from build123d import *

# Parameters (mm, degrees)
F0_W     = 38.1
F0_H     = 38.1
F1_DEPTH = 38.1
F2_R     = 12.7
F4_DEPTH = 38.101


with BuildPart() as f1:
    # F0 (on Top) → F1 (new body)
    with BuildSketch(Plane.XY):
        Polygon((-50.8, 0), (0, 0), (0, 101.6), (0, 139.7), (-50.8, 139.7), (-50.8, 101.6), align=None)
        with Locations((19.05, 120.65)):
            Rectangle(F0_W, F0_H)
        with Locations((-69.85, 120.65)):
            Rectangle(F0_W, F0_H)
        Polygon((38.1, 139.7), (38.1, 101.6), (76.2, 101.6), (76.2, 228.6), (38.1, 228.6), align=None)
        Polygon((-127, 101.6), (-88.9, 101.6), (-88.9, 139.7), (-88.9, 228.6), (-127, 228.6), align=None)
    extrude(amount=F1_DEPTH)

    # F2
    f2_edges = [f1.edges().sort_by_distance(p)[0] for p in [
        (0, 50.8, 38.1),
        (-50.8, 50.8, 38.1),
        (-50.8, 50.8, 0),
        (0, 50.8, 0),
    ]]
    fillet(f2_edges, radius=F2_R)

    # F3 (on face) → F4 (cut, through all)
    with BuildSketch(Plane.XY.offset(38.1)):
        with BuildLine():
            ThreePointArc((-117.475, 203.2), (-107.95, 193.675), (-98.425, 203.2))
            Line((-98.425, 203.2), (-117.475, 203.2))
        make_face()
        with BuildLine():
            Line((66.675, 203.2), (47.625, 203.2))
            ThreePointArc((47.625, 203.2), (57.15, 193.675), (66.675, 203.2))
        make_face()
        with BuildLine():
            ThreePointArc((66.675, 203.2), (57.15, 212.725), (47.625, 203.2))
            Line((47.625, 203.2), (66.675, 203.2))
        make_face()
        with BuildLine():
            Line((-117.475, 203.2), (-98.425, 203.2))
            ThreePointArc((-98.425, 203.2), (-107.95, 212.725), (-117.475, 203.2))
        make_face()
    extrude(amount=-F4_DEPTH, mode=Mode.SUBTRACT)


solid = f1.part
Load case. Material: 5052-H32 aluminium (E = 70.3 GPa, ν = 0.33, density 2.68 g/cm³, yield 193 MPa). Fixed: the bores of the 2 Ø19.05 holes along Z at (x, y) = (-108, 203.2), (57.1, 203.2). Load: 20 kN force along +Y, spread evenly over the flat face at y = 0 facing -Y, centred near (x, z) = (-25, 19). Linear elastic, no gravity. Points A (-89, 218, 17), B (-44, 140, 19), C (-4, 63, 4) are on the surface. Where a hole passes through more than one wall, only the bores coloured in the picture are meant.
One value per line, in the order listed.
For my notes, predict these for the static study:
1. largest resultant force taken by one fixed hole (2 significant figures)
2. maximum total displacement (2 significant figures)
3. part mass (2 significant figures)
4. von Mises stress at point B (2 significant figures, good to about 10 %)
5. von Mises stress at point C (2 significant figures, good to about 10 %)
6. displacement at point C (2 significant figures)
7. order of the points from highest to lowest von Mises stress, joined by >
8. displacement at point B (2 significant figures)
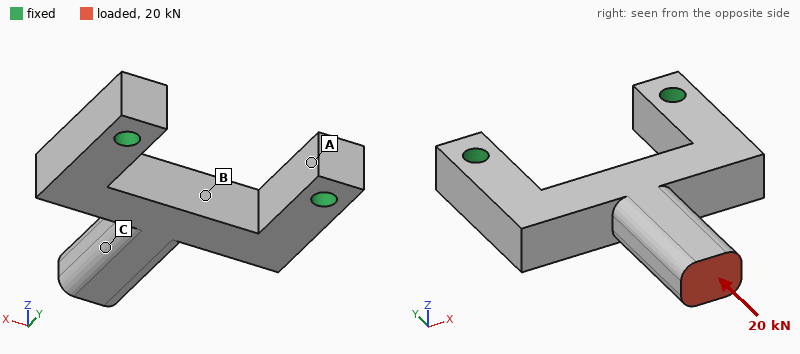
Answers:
11 kN
70 µm
1.9 kg
23 MPa
11 MPa
60 µm
B > C > A
51 µm
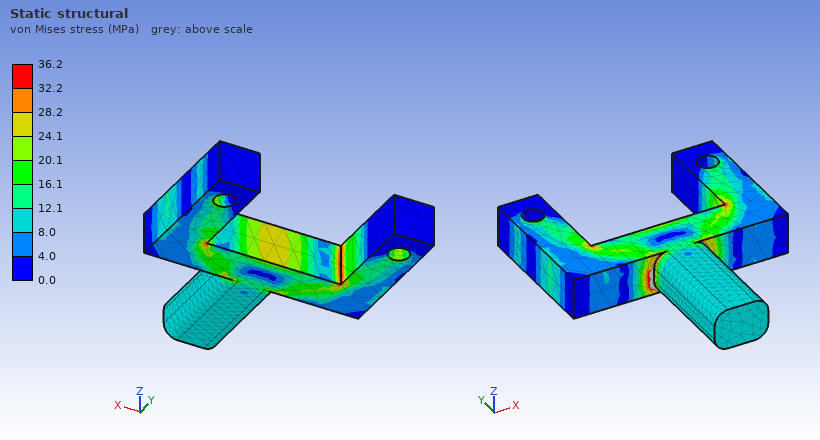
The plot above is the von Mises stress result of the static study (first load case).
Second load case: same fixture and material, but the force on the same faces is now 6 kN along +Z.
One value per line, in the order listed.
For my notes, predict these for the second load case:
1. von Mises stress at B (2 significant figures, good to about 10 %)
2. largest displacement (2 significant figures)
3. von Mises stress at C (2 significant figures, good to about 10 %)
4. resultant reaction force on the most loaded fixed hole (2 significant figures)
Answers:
28 MPa
1.1 mm
30 MPa
3.0 kN
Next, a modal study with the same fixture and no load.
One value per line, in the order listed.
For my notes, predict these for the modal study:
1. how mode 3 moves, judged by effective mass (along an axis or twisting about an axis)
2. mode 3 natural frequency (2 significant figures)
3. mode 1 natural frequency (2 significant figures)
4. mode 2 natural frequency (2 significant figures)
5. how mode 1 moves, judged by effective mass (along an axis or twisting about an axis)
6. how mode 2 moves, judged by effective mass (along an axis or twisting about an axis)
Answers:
along Z
2600 Hz
770 Hz
2000 Hz
along Z
along X
